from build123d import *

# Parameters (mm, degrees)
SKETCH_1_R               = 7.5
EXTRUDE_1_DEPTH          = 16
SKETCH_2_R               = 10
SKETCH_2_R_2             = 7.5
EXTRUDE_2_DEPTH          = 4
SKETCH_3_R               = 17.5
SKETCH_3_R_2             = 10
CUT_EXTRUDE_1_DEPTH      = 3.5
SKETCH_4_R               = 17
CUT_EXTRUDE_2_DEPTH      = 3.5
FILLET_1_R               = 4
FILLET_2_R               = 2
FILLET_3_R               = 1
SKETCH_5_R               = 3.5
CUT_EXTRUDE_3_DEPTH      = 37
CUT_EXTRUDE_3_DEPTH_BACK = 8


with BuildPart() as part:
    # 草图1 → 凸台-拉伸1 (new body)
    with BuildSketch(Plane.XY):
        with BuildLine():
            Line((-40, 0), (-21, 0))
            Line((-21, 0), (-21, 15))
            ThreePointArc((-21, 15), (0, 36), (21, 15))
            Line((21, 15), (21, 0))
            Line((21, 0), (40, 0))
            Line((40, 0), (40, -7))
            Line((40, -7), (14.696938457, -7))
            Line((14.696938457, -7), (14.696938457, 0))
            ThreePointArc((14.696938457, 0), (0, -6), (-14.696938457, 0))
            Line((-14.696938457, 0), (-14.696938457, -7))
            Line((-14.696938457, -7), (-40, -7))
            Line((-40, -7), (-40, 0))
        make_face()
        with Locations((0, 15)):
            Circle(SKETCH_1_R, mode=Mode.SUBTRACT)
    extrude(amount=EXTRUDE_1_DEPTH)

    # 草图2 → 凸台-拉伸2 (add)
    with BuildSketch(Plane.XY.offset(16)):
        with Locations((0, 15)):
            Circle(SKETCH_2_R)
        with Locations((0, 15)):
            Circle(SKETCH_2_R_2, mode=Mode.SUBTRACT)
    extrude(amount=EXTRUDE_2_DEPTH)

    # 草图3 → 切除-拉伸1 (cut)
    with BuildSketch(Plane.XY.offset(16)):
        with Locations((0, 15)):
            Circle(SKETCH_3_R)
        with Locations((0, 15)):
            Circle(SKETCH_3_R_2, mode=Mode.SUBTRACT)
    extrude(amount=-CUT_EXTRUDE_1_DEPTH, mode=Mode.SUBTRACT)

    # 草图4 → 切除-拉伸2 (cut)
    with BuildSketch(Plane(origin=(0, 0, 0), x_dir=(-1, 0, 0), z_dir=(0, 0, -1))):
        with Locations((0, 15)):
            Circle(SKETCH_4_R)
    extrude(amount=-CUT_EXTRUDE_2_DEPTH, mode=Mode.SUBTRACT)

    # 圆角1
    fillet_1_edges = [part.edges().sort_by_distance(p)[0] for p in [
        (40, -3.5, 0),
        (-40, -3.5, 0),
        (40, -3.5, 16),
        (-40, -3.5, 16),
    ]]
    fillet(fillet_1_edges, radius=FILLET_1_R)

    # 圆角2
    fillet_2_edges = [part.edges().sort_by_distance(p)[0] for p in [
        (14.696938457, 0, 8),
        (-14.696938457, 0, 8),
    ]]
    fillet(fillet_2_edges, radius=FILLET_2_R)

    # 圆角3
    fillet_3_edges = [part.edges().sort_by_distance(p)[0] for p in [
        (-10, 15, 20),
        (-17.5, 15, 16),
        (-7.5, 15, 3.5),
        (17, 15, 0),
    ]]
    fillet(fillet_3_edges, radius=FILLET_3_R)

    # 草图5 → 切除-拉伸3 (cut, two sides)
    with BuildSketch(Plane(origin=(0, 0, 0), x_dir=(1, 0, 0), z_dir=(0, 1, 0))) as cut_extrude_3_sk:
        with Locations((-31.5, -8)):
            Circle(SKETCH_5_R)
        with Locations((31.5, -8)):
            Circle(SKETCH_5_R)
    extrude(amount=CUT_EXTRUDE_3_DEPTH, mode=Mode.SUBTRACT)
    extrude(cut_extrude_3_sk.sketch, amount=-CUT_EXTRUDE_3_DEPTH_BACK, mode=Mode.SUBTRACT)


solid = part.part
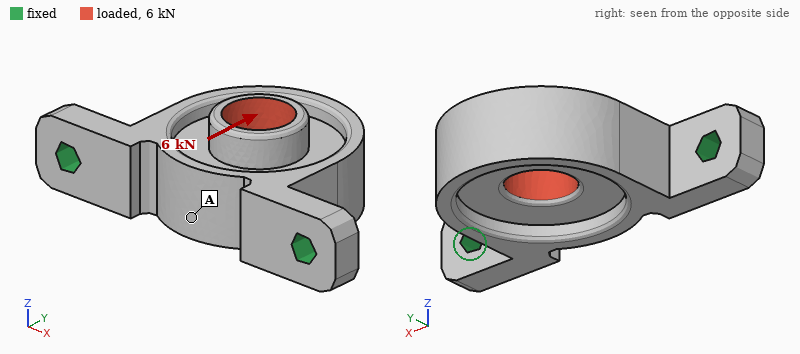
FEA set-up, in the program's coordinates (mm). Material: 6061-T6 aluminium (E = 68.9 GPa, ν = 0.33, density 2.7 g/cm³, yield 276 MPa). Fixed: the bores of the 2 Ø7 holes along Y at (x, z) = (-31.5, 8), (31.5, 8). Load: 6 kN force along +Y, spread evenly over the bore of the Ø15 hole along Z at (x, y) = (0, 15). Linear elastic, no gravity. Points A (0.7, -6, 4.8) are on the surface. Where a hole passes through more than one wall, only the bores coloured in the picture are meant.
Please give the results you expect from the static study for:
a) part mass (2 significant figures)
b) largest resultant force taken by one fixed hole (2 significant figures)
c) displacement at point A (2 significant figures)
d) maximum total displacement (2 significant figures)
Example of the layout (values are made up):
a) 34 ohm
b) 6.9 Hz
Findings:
a) 57 g
b) 3.7 kN
c) 0.032 mm
d) 0.18 mm
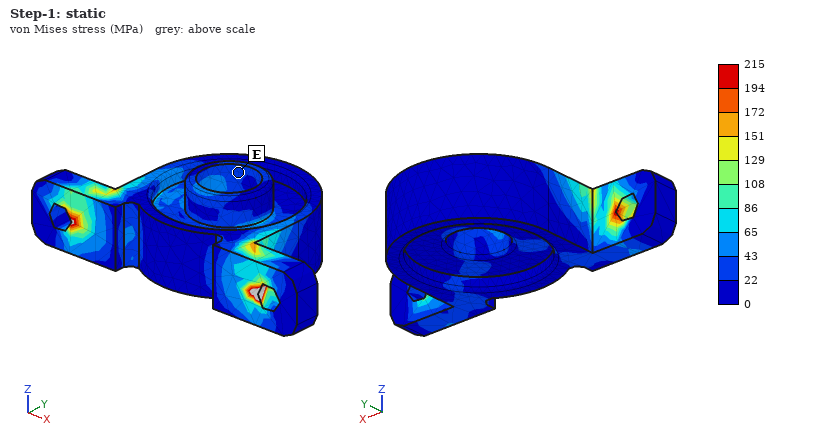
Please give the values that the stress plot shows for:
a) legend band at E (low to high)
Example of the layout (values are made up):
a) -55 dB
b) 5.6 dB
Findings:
a) 22 to 43 MPa
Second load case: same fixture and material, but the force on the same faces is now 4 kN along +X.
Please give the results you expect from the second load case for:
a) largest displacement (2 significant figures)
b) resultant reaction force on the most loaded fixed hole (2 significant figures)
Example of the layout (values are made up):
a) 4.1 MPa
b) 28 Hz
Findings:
a) 44 µm
b) 2.5 kN
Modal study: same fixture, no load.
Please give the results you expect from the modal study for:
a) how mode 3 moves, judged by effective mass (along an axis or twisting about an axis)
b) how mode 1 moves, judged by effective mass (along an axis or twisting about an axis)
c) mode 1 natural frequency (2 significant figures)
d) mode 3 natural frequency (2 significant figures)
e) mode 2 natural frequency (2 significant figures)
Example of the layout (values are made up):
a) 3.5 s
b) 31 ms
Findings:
a) twisting about Y
b) along Z
c) 2900 Hz
d) 9500 Hz
e) 9100 Hz
